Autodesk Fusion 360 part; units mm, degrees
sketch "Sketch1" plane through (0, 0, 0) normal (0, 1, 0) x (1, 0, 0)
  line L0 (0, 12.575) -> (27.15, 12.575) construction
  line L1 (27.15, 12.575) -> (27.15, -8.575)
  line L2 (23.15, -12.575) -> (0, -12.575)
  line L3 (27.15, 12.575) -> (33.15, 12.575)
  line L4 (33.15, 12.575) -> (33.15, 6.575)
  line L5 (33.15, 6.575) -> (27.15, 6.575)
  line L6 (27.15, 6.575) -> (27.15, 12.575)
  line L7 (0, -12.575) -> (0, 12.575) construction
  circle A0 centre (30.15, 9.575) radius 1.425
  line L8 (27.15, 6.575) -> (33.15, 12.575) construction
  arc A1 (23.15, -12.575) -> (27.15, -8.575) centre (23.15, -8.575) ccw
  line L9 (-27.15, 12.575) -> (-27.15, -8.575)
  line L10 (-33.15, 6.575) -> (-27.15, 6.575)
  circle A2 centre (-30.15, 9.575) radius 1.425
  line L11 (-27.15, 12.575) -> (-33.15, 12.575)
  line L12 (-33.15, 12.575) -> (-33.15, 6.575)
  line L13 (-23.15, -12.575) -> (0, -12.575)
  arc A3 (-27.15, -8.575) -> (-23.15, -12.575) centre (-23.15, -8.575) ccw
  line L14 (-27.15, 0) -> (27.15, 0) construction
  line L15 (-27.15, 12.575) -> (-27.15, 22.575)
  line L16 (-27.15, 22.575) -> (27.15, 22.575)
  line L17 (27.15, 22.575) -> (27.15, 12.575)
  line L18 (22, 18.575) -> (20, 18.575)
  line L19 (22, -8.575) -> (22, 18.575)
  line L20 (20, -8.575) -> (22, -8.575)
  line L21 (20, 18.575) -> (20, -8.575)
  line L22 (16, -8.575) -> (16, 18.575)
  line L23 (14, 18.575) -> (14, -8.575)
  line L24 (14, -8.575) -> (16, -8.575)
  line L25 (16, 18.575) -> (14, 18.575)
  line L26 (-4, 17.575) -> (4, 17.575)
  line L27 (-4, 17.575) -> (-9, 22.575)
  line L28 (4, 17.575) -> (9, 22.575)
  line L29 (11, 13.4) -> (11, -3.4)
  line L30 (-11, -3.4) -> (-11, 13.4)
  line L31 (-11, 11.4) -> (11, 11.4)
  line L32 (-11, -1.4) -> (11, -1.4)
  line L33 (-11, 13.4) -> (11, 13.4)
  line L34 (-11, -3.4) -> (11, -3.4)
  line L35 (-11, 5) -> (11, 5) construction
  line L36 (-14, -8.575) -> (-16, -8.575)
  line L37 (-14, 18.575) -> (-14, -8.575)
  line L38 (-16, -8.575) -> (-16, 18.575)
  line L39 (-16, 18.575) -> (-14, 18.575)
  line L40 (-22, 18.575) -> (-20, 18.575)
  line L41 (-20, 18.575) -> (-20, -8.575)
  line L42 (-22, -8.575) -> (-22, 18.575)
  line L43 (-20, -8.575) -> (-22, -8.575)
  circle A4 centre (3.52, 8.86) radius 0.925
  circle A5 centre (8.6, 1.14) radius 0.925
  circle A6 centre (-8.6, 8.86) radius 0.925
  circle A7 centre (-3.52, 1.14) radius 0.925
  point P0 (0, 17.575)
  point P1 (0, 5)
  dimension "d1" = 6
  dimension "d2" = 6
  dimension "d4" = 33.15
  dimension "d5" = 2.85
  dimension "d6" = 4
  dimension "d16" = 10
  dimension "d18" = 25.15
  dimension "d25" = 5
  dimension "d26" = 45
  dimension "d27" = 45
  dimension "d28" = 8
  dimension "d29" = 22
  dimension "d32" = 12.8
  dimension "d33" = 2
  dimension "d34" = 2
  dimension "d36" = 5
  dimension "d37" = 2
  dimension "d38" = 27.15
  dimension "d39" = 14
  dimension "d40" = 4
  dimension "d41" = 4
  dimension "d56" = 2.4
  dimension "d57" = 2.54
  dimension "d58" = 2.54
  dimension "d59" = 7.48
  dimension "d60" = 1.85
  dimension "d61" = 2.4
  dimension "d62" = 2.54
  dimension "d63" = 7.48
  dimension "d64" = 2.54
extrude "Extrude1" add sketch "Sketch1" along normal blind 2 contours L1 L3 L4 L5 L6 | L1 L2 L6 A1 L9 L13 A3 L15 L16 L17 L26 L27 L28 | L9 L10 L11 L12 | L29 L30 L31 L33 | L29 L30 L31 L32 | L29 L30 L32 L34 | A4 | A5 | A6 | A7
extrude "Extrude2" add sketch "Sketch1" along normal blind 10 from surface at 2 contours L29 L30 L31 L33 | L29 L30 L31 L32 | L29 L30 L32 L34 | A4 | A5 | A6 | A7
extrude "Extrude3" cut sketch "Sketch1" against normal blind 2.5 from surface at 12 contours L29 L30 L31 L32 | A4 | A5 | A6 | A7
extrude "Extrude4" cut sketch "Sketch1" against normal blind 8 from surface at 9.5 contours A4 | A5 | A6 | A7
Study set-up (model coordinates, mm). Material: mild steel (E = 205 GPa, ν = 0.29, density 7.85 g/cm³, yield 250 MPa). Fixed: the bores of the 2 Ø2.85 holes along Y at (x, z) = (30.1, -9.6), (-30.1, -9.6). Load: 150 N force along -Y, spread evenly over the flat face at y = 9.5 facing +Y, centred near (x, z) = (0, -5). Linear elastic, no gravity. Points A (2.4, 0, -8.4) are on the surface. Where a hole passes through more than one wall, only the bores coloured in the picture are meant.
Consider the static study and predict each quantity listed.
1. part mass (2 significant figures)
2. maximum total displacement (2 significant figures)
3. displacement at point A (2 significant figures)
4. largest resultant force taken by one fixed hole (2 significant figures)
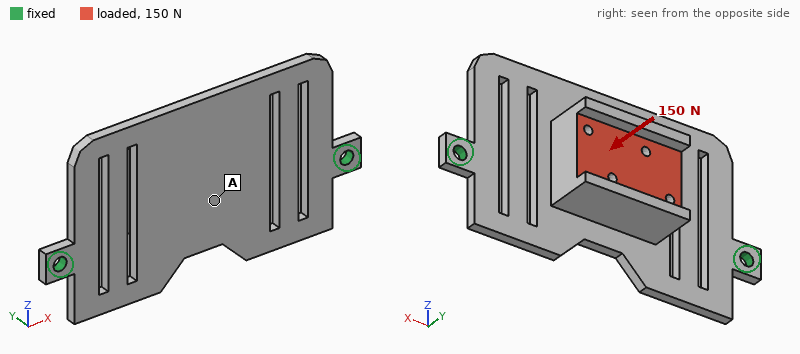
49 g
0.15 mm
0.084 mm
75 N
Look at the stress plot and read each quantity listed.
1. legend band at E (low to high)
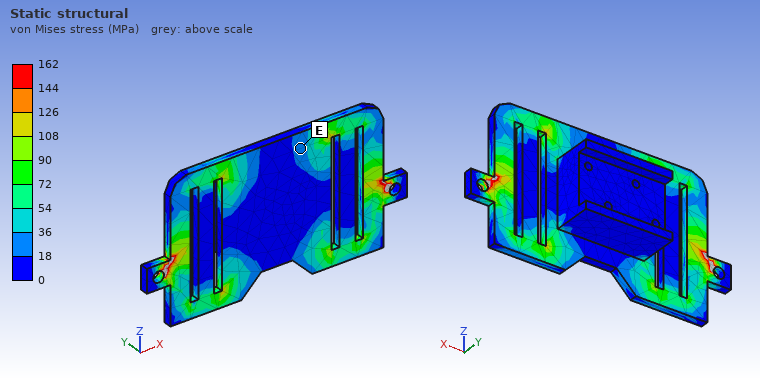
18 to 36 MPa
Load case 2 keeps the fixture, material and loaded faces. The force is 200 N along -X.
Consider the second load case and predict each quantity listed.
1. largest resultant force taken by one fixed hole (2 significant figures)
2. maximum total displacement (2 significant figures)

110 N
34 µm
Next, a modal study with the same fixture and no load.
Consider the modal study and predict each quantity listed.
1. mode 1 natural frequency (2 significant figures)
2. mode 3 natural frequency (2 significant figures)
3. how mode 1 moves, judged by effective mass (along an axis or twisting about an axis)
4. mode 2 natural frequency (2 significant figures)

900 Hz
2500 Hz
along Y
1600 Hz
